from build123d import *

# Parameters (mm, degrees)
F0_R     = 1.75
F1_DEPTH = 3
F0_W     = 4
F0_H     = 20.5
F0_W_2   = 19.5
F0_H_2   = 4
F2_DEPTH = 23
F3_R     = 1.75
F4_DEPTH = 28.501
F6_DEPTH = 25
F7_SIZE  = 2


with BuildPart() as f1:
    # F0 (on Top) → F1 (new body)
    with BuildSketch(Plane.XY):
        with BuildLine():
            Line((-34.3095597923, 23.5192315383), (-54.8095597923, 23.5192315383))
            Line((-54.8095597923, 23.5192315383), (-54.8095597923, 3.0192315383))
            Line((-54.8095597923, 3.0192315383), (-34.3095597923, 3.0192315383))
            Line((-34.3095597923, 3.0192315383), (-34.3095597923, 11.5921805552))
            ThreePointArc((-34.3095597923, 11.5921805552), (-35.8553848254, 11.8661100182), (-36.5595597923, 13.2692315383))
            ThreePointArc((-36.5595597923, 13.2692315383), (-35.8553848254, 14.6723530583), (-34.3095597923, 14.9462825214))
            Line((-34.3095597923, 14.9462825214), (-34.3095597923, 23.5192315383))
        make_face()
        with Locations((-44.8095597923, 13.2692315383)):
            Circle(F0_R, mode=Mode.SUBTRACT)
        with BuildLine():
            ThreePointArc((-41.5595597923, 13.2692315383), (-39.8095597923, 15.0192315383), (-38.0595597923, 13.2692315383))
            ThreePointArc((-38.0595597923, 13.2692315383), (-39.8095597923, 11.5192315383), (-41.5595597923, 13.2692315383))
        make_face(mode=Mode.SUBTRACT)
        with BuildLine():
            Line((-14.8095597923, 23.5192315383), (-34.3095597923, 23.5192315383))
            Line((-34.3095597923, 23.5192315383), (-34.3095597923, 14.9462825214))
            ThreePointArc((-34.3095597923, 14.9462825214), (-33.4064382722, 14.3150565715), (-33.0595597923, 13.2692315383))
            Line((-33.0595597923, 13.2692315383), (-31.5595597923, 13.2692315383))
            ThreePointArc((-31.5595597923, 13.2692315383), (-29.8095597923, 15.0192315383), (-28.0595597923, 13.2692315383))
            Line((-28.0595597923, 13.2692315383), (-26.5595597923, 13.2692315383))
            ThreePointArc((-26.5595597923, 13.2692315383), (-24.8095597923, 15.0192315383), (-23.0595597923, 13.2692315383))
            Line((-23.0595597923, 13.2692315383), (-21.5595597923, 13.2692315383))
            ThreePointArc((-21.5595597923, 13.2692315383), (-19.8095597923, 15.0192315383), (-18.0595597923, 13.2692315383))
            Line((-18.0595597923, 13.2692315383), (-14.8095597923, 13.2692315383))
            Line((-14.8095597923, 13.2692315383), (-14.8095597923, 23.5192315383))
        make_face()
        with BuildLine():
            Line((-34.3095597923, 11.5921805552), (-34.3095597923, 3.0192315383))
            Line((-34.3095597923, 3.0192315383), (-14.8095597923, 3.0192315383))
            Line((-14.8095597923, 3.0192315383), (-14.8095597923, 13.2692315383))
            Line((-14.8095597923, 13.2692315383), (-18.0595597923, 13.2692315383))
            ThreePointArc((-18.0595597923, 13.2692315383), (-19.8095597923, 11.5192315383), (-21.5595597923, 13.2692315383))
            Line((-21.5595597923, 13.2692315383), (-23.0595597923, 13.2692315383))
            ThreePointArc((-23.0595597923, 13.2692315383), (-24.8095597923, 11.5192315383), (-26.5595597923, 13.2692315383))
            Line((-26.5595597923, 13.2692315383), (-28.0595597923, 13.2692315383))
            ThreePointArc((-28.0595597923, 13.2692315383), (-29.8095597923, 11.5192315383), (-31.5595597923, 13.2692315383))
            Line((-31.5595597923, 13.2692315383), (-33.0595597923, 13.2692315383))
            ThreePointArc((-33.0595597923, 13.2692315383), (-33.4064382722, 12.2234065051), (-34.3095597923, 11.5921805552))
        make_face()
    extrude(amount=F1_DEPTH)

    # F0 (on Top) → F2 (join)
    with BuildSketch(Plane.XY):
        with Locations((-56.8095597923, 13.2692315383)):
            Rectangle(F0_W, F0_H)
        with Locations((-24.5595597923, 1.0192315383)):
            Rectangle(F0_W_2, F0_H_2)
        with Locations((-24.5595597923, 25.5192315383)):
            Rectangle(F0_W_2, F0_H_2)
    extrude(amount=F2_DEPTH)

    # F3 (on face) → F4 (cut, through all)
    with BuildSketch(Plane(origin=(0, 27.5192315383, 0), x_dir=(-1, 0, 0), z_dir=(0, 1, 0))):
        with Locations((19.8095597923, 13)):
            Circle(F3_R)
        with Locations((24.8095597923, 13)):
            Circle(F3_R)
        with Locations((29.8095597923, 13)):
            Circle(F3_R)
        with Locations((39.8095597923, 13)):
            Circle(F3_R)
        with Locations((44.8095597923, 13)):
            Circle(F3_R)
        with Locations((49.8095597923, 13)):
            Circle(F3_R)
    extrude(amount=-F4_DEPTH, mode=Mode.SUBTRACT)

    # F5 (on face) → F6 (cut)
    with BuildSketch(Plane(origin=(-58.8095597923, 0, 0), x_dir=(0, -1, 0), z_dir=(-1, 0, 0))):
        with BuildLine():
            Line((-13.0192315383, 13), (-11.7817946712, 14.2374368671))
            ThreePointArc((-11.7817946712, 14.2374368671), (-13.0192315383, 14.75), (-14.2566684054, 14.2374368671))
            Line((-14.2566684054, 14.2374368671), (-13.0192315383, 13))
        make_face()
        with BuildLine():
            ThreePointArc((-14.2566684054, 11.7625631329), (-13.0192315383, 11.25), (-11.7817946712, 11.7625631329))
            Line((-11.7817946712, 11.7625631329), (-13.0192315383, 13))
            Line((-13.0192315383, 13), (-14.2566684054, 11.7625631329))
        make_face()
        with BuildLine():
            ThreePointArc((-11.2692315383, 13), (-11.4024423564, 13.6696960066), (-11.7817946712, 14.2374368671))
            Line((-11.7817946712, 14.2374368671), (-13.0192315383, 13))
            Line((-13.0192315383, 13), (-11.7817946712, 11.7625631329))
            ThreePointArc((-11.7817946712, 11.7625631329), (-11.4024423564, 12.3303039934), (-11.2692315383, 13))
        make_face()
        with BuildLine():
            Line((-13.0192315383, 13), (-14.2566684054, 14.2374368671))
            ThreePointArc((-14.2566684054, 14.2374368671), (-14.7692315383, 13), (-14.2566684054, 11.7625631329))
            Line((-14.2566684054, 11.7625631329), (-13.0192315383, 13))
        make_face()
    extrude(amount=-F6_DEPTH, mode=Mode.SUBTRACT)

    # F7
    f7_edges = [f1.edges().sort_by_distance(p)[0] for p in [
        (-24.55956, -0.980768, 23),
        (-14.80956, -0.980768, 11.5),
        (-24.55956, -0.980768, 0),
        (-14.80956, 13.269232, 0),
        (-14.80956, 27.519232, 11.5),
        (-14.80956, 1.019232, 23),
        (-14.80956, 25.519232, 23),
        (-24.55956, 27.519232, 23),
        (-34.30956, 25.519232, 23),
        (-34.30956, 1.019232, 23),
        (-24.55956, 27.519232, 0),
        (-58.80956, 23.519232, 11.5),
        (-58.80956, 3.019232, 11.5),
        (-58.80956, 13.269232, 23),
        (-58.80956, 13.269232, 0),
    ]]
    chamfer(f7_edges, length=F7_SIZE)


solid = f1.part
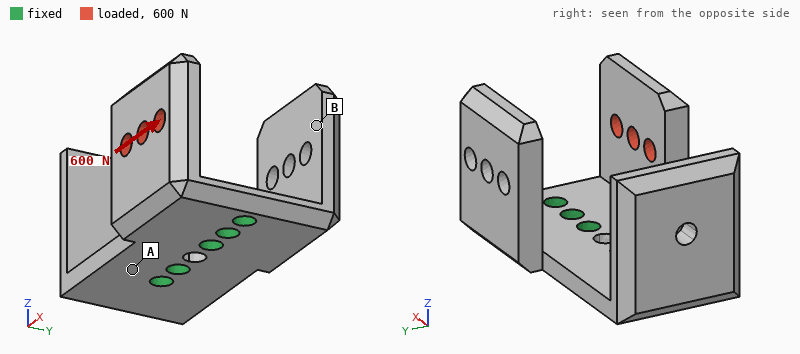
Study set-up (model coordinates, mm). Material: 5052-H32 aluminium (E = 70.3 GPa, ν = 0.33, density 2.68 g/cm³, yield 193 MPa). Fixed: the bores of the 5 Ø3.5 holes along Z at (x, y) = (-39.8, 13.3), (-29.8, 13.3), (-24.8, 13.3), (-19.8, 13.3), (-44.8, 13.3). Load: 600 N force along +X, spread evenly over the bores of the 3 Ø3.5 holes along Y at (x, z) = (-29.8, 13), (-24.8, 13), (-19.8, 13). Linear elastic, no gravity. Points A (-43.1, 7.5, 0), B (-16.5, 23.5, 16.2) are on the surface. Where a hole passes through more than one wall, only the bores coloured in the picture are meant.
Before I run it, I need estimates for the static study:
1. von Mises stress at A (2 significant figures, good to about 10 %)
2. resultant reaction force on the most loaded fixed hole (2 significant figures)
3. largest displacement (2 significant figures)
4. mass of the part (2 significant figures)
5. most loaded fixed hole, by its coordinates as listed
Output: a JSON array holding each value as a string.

["43 MPa", "490 N", "0.15 mm", "19 g", "(-19.8, 13.3)"]
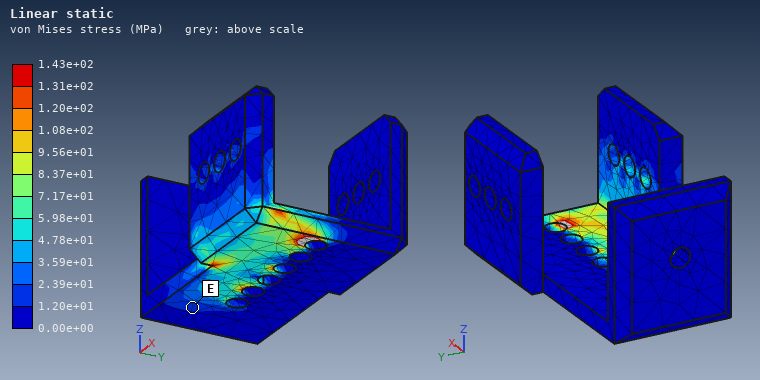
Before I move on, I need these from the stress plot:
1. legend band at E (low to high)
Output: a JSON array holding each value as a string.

["1.20e+01 to 2.39e+01 MPa"]
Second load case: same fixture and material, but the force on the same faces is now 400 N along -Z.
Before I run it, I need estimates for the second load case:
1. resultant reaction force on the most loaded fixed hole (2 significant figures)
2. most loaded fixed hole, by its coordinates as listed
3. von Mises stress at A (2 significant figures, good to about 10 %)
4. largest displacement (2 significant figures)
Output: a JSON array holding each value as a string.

["150 N", "(-19.8, 13.3)", "27 MPa", "0.15 mm"]
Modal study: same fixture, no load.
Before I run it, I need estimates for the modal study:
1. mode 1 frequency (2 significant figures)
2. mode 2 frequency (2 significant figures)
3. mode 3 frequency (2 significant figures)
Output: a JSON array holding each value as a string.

["2800 Hz", "3300 Hz", "3300 Hz"]
